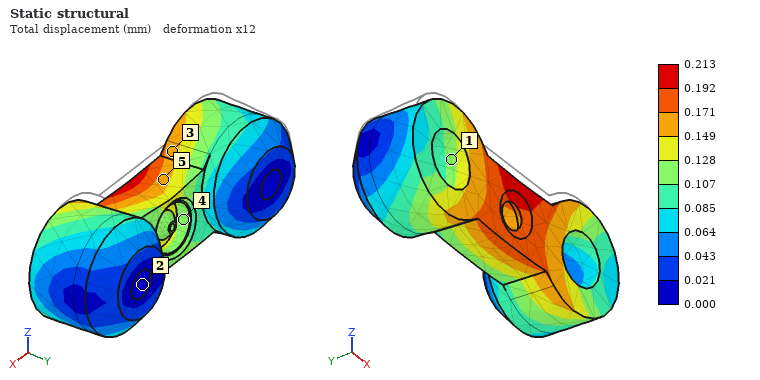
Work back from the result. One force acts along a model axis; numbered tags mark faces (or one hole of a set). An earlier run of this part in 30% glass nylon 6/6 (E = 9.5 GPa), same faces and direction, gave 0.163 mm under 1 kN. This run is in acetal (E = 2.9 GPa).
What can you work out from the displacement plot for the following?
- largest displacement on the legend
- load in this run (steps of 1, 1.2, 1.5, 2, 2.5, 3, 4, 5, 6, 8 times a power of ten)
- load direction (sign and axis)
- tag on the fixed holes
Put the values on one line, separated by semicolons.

0.213 mm; 400 N; -Z; 2
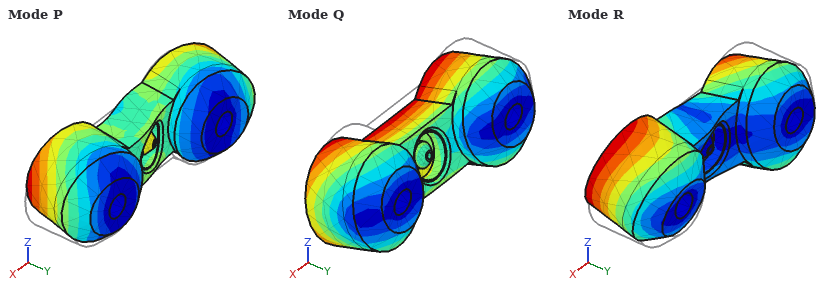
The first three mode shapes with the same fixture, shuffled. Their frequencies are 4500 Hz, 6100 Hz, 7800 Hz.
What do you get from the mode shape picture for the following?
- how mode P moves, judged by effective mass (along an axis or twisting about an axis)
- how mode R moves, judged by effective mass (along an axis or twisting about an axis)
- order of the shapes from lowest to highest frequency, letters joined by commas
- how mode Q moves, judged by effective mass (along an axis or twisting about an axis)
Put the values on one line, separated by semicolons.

along X; twisting about Y; Q, R, P; along Z
